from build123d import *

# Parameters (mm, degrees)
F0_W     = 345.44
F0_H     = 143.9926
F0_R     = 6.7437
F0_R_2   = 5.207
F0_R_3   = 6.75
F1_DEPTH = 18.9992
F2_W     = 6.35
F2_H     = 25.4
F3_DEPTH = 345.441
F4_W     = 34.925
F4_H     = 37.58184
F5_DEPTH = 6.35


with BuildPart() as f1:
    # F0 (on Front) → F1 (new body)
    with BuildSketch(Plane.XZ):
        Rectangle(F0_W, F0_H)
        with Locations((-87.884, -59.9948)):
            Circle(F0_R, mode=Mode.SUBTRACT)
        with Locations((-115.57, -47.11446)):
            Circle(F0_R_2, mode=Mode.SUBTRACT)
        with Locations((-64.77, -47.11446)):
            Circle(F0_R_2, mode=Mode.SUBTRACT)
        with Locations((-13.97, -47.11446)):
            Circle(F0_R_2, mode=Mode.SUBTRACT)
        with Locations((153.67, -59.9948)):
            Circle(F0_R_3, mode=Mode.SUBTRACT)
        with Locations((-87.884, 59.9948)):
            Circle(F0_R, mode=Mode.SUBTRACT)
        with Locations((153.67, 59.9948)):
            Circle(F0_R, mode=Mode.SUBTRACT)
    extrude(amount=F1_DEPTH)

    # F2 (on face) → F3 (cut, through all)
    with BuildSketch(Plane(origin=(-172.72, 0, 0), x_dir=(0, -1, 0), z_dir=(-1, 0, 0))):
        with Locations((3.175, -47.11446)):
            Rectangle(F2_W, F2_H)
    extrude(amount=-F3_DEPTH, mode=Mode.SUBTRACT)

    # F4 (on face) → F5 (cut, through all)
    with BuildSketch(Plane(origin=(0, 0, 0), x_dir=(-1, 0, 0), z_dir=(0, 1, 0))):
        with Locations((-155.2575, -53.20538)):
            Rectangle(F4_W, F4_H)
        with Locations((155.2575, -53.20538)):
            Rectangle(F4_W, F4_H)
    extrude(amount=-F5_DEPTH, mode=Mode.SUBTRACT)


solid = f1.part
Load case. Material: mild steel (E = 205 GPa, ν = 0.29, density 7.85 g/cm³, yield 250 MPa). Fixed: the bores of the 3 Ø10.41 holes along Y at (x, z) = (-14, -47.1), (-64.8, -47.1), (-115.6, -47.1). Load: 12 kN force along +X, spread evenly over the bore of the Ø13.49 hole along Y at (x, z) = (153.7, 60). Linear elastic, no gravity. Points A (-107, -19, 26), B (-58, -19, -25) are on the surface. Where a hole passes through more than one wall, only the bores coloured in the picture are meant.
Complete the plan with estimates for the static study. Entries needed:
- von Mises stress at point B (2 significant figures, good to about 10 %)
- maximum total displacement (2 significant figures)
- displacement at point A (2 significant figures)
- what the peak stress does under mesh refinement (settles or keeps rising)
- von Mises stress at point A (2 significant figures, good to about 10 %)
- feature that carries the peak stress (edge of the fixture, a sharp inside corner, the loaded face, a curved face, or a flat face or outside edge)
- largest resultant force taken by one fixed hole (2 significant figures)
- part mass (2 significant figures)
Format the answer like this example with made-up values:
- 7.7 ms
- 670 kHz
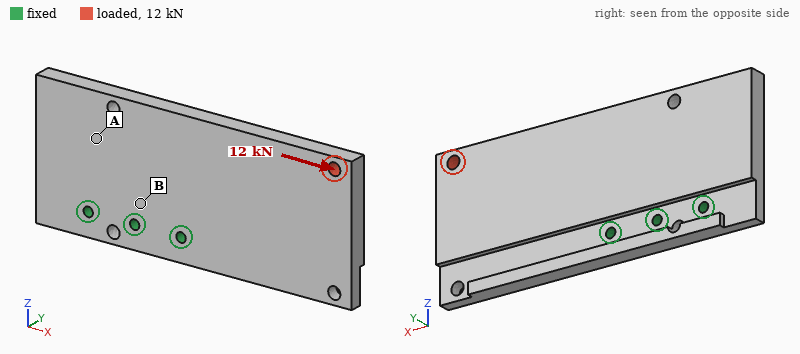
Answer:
- 17 MPa
- 59 µm
- 10 µm
- keeps rising
- 7.3 MPa
- edge of the fixture
- 13 kN
- 6.8 kg
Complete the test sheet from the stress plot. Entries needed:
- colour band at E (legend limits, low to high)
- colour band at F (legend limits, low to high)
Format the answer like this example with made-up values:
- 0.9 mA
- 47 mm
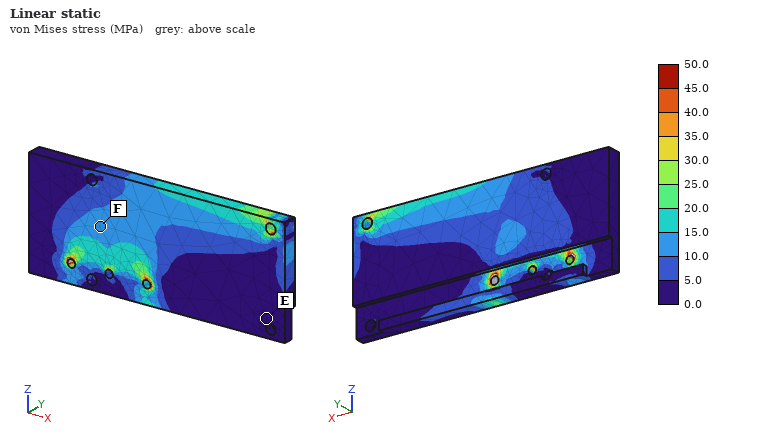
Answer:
- 0.0 to 5.0 MPa
- 10.0 to 15.0 MPa
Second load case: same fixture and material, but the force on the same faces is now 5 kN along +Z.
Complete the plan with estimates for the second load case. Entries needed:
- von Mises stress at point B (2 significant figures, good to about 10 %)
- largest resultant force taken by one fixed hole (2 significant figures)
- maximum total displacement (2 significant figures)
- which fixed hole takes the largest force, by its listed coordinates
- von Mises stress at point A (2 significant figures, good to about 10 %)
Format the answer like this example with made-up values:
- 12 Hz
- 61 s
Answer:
- 11 MPa
- 13 kN
- 56 µm
- (-14, -47.1)
- 5.9 MPa
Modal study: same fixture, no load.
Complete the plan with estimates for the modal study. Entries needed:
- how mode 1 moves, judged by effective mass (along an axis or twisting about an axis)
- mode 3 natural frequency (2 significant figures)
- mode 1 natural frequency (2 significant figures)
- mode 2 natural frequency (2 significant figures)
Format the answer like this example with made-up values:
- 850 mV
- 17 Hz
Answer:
- along Y
- 1100 Hz
- 310 Hz
- 620 Hz
